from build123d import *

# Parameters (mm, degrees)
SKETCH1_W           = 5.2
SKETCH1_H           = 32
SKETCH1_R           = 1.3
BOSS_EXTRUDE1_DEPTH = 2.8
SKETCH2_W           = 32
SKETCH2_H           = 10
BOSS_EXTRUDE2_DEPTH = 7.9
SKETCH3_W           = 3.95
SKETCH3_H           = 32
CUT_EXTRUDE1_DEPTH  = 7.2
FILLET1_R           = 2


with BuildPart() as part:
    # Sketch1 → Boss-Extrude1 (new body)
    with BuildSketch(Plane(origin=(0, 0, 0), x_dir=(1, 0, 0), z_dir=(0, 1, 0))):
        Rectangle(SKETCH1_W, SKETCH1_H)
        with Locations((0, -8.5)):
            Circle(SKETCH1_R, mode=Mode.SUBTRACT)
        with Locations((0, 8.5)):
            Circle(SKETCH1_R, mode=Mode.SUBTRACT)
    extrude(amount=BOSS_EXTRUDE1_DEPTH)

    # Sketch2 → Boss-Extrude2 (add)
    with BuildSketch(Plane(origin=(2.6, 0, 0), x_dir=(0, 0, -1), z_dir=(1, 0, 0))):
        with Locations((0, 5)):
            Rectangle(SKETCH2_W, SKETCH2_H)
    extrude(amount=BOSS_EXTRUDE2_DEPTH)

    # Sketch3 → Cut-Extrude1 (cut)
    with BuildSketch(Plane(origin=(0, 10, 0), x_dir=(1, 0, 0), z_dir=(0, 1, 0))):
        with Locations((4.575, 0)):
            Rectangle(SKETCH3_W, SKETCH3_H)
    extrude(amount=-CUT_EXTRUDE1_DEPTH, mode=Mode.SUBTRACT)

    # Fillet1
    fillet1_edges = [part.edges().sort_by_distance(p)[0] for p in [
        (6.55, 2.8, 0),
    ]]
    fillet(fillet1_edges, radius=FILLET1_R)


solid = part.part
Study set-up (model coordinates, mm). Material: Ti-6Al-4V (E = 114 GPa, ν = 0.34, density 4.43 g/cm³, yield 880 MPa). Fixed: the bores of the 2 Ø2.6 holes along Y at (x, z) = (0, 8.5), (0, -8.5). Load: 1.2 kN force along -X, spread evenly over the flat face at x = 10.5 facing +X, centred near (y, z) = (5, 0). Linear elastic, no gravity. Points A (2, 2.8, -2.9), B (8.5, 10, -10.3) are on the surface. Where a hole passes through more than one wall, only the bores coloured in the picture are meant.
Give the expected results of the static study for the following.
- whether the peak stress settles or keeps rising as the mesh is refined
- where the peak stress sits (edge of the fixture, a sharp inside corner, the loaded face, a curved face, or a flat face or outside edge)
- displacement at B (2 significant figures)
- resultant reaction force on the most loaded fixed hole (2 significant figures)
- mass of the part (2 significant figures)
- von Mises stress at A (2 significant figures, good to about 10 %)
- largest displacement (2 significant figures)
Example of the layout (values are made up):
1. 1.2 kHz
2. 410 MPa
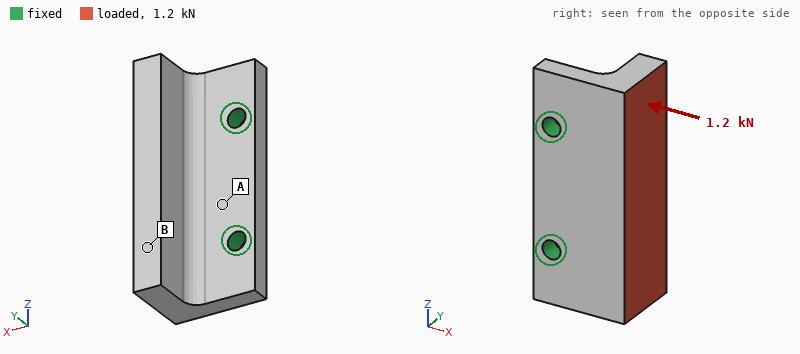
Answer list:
1. keeps rising
2. edge of the fixture
3. 51 µm
4. 600 N
5. 9.2 g
6. 69 MPa
7. 57 µm
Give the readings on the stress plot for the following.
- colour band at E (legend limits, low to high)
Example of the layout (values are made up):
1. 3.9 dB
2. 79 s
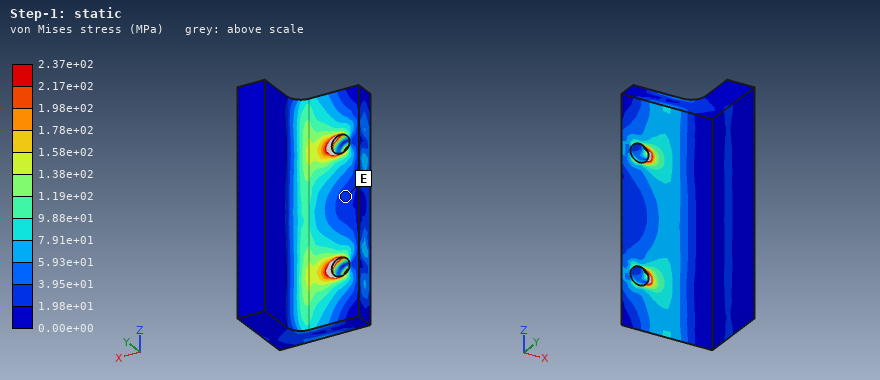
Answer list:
1. 1.98e+01 to 3.95e+01 MPa
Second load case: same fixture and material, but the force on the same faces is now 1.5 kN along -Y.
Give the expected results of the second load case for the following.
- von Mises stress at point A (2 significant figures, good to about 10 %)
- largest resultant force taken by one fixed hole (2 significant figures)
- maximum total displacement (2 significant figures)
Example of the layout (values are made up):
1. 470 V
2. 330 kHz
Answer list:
1. 160 MPa
2. 750 N
3. 0.15 mm
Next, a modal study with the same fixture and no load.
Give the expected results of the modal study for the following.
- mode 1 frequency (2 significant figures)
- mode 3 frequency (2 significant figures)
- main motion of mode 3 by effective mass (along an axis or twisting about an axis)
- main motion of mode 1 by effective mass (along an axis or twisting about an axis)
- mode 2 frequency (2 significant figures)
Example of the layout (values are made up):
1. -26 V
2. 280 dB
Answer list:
1. 8300 Hz
2. 26 kHz
3. along Z
4. along Y
5. 14 kHz
